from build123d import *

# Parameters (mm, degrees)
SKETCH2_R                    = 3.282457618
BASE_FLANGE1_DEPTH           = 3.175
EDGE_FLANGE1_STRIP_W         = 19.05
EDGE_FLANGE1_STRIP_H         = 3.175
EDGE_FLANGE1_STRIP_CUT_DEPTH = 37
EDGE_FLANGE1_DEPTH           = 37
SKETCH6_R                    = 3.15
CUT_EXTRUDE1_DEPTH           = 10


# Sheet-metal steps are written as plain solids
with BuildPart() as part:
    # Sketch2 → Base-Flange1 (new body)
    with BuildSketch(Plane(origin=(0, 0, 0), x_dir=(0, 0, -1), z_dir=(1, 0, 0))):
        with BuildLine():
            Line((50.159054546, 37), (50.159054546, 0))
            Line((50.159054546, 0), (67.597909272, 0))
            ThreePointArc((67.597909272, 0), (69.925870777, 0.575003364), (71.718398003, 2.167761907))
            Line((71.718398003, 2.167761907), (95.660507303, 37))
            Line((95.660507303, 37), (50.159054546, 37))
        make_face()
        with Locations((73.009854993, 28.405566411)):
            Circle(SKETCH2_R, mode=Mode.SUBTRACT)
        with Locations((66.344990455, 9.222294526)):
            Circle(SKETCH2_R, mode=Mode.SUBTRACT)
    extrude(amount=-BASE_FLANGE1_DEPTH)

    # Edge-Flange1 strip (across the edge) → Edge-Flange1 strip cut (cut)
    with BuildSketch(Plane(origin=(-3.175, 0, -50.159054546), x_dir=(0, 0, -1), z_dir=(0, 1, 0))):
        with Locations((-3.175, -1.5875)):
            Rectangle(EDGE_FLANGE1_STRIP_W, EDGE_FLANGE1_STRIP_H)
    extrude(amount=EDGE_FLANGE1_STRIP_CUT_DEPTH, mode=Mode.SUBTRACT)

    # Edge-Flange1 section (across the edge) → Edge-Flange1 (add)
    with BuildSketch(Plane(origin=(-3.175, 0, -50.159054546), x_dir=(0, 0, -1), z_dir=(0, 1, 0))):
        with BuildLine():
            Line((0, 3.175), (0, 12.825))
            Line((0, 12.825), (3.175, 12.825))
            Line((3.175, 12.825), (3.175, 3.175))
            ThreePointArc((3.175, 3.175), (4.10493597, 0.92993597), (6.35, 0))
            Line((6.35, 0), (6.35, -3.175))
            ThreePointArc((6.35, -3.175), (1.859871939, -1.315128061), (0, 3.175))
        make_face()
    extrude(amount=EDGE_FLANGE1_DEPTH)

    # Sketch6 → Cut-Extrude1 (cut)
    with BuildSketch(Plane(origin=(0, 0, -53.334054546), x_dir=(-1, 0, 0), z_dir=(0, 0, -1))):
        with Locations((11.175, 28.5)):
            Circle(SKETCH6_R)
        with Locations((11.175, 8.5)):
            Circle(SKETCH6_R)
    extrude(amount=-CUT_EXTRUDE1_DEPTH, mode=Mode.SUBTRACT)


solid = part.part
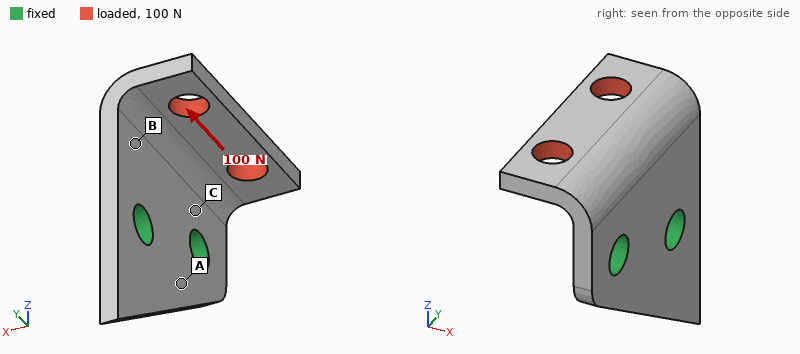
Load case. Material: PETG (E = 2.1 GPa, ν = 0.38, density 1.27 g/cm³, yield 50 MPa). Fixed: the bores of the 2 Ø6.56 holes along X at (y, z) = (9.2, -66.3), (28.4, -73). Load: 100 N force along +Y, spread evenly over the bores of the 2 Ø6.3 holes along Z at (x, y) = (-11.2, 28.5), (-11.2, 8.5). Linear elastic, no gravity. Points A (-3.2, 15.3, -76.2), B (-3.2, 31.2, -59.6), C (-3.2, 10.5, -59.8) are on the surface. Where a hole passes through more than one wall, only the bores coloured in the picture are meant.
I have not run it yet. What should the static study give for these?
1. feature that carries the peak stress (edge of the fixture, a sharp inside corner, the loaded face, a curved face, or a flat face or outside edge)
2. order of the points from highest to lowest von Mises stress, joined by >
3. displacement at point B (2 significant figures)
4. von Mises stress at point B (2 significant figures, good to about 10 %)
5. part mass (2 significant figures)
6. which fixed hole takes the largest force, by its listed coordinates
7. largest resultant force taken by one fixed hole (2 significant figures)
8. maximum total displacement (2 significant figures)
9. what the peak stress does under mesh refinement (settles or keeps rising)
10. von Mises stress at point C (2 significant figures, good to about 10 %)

edge of the fixture
C > B > A
0.20 mm
5.9 MPa
6.0 g
(9.2, -66.3)
100 N
0.70 mm
keeps rising
8.8 MPa
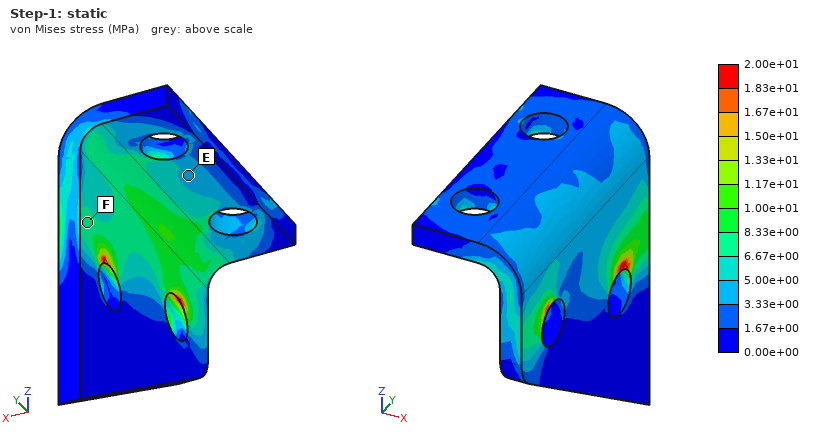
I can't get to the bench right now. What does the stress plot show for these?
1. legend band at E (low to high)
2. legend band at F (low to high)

3.33e+00 to 5.00e+00 MPa
6.67e+00 to 8.33e+00 MPa
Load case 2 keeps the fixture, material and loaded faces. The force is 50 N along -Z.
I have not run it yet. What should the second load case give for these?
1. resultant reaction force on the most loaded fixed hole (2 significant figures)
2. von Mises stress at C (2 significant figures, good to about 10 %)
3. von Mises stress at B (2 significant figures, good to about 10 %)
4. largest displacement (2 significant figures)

27 N
9.9 MPa
6.4 MPa
0.63 mm
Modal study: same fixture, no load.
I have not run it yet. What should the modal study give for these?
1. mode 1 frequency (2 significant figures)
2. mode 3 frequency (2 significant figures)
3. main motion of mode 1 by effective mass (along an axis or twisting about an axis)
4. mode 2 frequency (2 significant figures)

1100 Hz
2500 Hz
along X
1800 Hz
